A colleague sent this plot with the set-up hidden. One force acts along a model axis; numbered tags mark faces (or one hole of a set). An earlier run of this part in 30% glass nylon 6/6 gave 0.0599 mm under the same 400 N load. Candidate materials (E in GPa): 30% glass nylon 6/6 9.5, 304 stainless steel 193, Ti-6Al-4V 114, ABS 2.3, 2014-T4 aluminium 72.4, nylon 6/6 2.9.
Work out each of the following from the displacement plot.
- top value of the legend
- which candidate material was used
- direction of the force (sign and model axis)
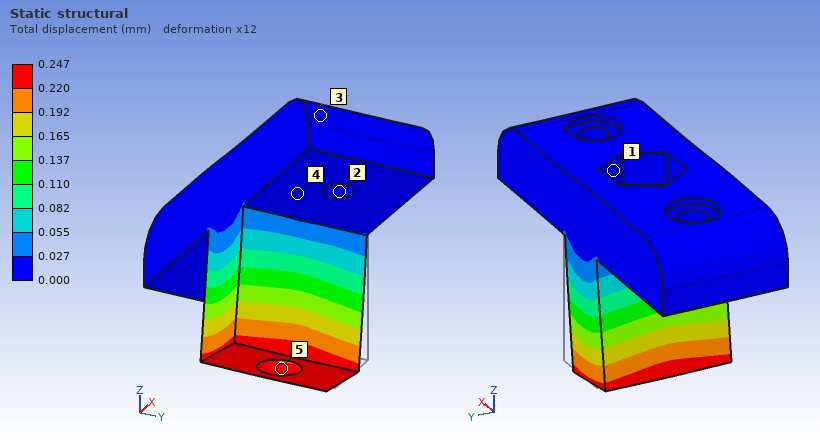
0.247 mm
ABS
-X
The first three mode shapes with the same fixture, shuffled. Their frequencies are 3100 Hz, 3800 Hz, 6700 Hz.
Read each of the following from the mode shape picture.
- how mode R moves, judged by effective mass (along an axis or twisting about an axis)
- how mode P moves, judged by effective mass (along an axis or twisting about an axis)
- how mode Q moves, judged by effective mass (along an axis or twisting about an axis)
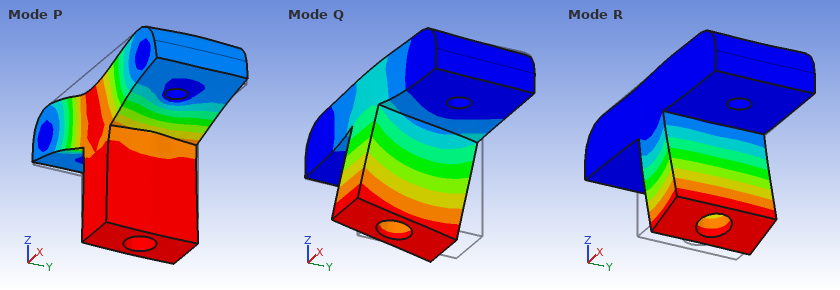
along X
along Z
along Y
